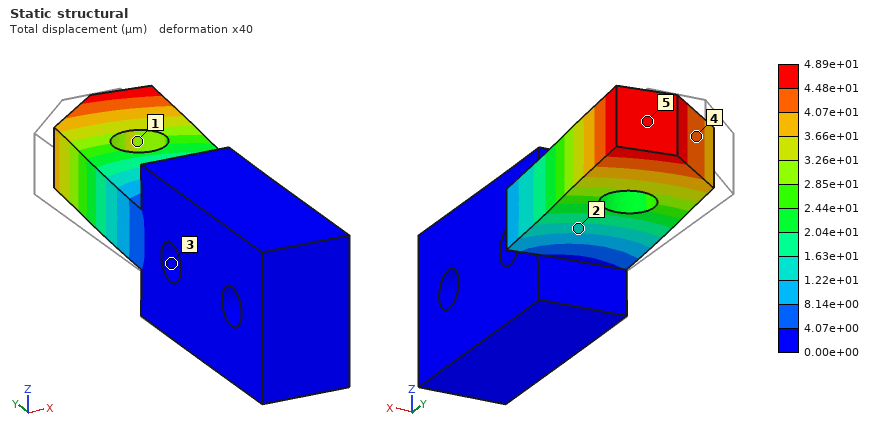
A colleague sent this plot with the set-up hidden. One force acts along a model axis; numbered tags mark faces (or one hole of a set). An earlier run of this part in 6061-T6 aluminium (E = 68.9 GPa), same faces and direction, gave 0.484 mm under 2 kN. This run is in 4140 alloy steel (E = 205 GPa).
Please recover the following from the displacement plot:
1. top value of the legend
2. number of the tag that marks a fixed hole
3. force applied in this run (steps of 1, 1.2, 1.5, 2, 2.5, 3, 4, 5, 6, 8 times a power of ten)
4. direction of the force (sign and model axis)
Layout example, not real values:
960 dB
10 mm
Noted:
4.89e+01 µm
3
600 N
+X
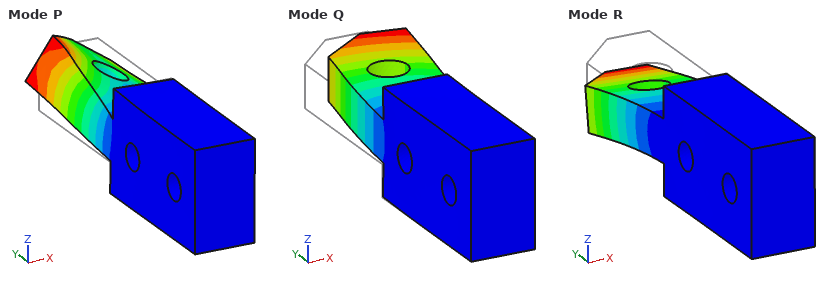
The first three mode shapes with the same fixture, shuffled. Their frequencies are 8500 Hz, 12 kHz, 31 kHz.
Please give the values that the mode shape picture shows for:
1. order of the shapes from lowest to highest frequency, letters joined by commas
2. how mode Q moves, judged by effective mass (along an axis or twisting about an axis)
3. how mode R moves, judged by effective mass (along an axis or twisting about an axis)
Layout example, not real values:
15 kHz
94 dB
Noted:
R, Q, P
along X
along Z
